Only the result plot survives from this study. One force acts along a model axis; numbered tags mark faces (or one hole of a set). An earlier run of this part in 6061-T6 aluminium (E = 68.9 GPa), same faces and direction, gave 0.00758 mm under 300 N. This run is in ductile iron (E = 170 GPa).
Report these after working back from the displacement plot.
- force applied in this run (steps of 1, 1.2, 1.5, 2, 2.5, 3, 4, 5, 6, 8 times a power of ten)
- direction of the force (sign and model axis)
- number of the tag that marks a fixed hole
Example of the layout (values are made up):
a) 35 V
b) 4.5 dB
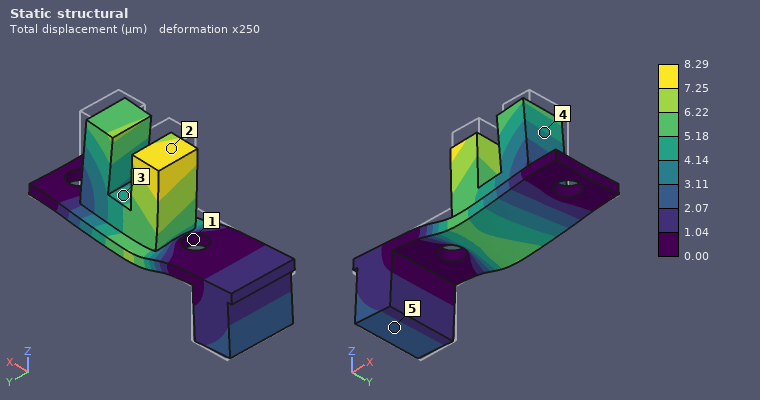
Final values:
a) 800 N
b) -Z
c) 1
